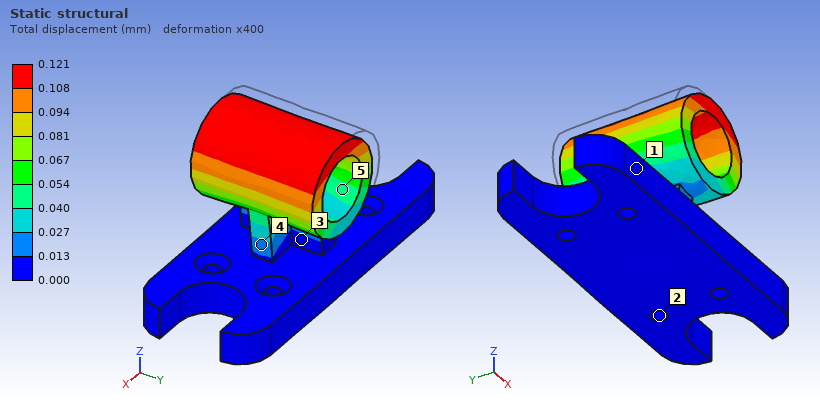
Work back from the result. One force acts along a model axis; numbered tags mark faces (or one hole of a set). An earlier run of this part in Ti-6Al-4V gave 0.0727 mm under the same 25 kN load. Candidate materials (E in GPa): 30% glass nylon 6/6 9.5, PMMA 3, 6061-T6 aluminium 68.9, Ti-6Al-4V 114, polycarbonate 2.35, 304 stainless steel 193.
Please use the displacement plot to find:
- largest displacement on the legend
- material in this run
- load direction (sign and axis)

0.121 mm
6061-T6 aluminium
+X
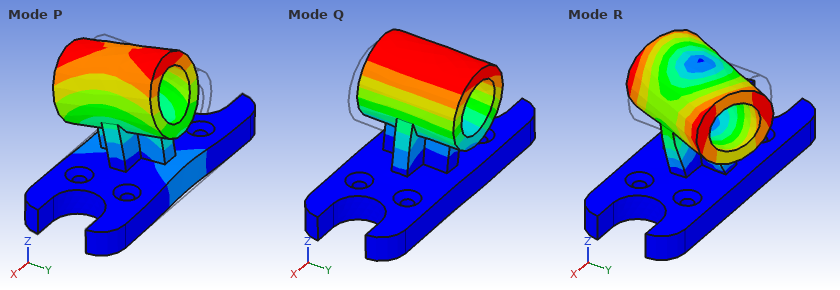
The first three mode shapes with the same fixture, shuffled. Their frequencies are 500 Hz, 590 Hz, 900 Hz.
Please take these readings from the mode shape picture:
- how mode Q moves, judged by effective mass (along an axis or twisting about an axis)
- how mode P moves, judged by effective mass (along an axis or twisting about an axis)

along X
along Y
